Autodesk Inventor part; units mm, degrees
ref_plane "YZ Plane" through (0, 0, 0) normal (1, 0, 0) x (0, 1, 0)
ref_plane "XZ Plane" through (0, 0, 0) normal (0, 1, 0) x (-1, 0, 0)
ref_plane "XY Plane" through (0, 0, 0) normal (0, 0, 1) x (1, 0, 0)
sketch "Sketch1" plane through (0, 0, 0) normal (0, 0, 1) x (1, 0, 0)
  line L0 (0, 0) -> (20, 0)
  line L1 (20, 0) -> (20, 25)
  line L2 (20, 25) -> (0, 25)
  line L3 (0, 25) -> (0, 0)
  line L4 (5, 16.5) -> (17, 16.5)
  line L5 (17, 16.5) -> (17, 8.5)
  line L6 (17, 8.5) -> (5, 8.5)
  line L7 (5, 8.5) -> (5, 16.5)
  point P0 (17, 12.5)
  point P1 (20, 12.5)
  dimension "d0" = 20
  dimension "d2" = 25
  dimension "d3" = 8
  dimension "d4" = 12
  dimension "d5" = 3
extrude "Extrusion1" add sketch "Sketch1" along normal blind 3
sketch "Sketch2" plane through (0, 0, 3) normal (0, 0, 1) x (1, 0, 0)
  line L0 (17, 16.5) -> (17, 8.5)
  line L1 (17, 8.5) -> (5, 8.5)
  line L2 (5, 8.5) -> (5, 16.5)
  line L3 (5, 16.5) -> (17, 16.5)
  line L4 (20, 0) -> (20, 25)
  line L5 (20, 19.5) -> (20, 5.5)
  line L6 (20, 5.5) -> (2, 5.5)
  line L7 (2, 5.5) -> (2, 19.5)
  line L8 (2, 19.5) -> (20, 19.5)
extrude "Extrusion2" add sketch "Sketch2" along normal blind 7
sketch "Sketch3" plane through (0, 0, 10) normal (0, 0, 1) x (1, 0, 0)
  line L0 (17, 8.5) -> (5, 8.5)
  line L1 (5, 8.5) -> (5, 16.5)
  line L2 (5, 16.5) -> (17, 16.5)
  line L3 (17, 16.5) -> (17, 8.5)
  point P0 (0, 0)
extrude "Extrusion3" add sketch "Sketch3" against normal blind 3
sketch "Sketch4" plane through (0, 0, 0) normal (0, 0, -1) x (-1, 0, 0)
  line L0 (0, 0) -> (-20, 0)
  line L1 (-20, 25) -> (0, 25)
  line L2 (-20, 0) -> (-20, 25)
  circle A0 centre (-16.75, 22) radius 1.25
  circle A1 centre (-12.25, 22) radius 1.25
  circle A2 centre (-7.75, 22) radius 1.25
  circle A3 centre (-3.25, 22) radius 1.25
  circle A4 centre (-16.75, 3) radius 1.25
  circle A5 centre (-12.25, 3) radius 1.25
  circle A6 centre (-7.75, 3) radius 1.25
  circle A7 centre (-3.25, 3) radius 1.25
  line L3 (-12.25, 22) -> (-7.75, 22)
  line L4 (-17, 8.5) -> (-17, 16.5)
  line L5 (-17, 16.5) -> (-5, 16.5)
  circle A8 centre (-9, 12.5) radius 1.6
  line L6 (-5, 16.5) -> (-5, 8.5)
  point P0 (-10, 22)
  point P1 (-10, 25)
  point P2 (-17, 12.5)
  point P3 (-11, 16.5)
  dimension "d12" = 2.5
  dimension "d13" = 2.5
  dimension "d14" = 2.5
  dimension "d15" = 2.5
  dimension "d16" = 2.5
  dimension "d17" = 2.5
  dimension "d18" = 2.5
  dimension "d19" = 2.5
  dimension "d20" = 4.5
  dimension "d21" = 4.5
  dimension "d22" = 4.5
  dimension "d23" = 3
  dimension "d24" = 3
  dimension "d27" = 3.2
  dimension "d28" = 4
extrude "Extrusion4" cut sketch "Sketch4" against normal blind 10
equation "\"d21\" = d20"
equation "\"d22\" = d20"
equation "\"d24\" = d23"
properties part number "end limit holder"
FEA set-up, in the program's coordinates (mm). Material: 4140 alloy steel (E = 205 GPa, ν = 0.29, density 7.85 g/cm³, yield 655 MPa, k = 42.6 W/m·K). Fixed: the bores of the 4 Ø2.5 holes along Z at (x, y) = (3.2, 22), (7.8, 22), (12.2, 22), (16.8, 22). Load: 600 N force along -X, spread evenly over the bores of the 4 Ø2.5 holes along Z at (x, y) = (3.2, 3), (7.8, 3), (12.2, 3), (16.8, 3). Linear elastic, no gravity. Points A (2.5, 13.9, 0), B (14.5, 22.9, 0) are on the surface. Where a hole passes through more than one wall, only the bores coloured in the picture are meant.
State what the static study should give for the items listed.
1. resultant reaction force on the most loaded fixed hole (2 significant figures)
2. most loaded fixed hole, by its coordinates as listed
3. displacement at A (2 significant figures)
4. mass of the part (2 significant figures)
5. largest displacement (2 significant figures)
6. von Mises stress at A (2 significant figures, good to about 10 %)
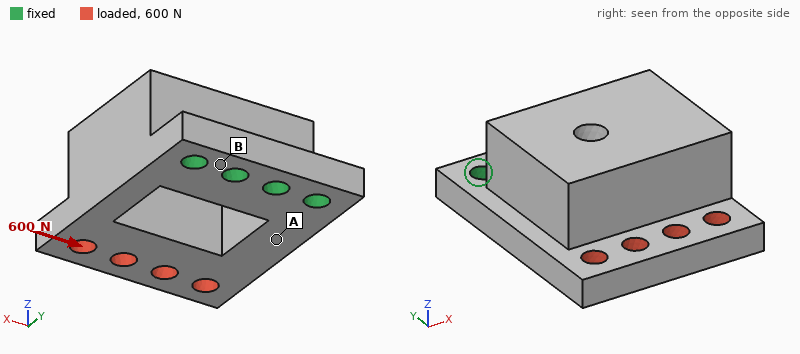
770 N
(3.2, 22)
6.1 µm
19 g
21 µm
67 MPa
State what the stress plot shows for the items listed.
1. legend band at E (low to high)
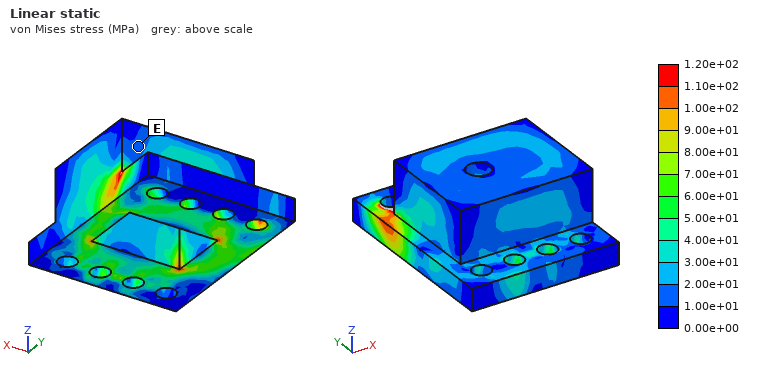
1.00e+01 to 2.00e+01 MPa
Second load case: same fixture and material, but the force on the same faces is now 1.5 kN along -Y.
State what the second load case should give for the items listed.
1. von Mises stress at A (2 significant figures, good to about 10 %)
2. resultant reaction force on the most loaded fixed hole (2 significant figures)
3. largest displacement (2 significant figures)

60 MPa
700 N
14 µm
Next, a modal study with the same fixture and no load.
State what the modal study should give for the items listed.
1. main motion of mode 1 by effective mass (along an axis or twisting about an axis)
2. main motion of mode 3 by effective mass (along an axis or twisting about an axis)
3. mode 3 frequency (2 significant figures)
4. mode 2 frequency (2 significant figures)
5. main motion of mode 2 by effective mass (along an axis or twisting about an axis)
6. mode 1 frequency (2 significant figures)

along Z
along X
21 kHz
12 kHz
along X
5300 Hz
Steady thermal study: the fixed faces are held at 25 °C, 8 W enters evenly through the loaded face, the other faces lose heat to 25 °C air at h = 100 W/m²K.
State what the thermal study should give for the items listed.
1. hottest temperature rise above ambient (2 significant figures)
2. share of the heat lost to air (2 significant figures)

44 K
41 %
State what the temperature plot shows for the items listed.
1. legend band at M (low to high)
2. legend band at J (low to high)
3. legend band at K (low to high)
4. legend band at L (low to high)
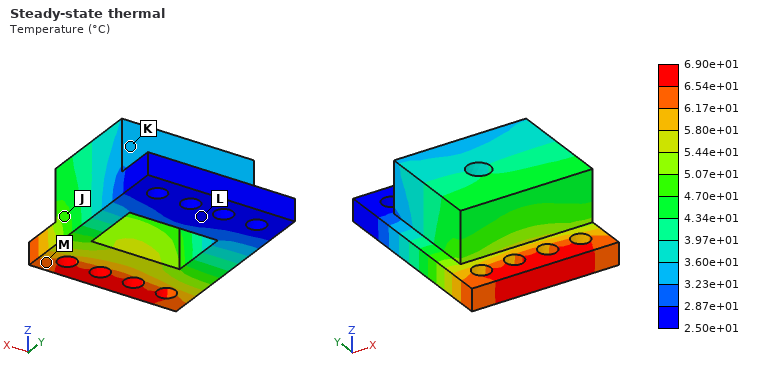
6.17e+01 to 6.54e+01 °C
4.70e+01 to 5.07e+01 °C
3.23e+01 to 3.60e+01 °C
2.50e+01 to 2.87e+01 °C
